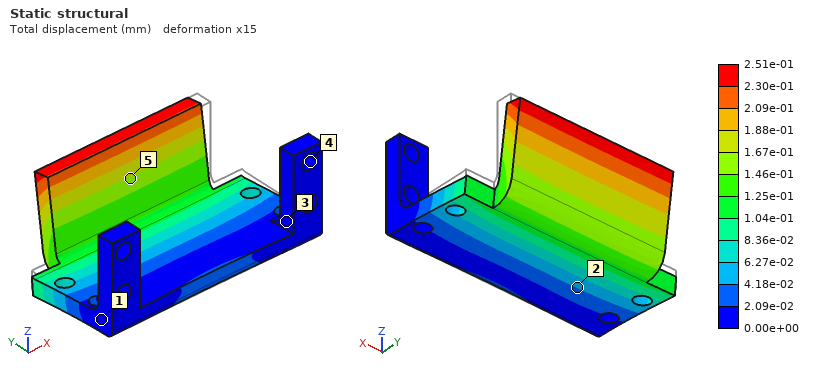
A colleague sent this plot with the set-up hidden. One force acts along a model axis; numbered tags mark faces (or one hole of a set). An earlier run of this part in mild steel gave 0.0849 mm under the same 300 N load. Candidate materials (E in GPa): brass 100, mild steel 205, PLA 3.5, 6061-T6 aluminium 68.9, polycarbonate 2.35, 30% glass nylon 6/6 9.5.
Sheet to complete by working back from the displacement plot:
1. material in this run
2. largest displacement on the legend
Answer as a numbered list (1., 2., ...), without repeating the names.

1. 6061-T6 aluminium
2. 2.51e-01 mm
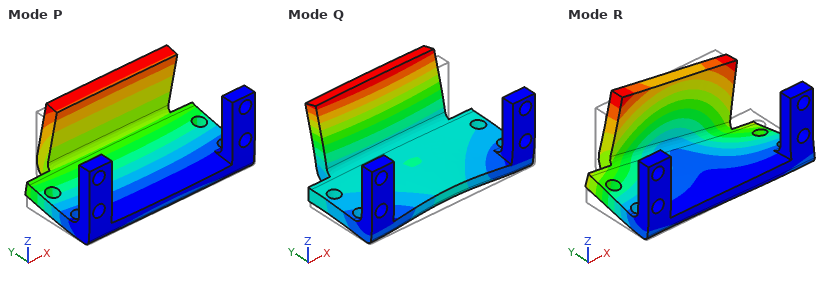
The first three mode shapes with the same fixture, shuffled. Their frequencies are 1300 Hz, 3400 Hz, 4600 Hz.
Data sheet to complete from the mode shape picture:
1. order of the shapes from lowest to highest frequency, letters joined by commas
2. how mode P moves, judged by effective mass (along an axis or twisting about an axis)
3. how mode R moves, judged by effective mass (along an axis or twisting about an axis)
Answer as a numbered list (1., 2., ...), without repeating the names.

1. P, R, Q
2. along Z
3. along X
